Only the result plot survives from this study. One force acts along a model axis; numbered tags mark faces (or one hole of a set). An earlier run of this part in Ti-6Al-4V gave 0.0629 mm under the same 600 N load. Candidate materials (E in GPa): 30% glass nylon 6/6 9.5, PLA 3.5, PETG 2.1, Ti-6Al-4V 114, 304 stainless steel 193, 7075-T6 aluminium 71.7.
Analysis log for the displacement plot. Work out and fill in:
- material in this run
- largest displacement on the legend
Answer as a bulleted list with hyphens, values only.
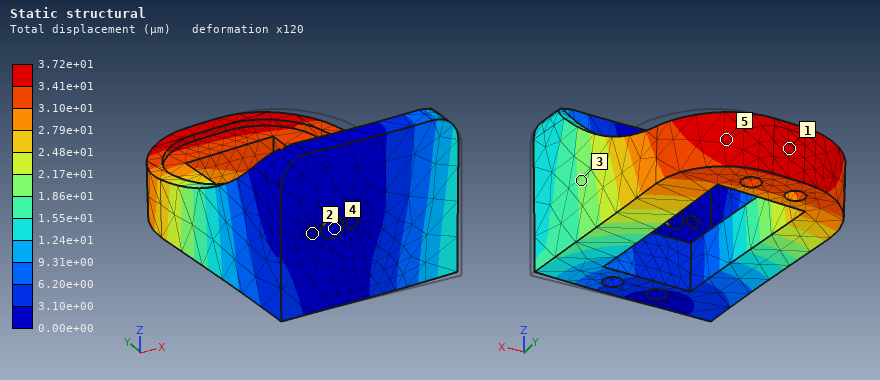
- 304 stainless steel
- 3.72e+01 µm
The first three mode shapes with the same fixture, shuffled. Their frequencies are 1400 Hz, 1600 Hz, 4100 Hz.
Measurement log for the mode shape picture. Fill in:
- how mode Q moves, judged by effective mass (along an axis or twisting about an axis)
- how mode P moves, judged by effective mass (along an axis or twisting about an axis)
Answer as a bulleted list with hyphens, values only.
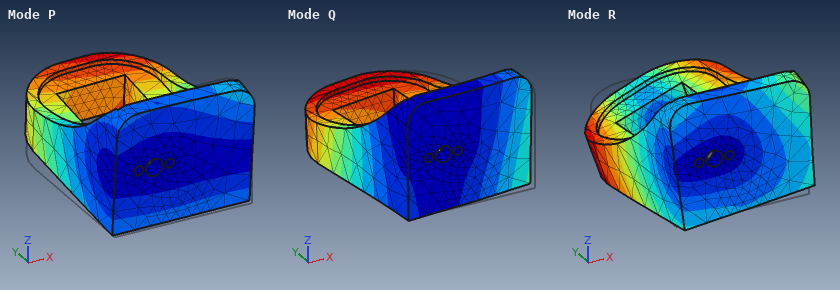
- along X
- along Z
